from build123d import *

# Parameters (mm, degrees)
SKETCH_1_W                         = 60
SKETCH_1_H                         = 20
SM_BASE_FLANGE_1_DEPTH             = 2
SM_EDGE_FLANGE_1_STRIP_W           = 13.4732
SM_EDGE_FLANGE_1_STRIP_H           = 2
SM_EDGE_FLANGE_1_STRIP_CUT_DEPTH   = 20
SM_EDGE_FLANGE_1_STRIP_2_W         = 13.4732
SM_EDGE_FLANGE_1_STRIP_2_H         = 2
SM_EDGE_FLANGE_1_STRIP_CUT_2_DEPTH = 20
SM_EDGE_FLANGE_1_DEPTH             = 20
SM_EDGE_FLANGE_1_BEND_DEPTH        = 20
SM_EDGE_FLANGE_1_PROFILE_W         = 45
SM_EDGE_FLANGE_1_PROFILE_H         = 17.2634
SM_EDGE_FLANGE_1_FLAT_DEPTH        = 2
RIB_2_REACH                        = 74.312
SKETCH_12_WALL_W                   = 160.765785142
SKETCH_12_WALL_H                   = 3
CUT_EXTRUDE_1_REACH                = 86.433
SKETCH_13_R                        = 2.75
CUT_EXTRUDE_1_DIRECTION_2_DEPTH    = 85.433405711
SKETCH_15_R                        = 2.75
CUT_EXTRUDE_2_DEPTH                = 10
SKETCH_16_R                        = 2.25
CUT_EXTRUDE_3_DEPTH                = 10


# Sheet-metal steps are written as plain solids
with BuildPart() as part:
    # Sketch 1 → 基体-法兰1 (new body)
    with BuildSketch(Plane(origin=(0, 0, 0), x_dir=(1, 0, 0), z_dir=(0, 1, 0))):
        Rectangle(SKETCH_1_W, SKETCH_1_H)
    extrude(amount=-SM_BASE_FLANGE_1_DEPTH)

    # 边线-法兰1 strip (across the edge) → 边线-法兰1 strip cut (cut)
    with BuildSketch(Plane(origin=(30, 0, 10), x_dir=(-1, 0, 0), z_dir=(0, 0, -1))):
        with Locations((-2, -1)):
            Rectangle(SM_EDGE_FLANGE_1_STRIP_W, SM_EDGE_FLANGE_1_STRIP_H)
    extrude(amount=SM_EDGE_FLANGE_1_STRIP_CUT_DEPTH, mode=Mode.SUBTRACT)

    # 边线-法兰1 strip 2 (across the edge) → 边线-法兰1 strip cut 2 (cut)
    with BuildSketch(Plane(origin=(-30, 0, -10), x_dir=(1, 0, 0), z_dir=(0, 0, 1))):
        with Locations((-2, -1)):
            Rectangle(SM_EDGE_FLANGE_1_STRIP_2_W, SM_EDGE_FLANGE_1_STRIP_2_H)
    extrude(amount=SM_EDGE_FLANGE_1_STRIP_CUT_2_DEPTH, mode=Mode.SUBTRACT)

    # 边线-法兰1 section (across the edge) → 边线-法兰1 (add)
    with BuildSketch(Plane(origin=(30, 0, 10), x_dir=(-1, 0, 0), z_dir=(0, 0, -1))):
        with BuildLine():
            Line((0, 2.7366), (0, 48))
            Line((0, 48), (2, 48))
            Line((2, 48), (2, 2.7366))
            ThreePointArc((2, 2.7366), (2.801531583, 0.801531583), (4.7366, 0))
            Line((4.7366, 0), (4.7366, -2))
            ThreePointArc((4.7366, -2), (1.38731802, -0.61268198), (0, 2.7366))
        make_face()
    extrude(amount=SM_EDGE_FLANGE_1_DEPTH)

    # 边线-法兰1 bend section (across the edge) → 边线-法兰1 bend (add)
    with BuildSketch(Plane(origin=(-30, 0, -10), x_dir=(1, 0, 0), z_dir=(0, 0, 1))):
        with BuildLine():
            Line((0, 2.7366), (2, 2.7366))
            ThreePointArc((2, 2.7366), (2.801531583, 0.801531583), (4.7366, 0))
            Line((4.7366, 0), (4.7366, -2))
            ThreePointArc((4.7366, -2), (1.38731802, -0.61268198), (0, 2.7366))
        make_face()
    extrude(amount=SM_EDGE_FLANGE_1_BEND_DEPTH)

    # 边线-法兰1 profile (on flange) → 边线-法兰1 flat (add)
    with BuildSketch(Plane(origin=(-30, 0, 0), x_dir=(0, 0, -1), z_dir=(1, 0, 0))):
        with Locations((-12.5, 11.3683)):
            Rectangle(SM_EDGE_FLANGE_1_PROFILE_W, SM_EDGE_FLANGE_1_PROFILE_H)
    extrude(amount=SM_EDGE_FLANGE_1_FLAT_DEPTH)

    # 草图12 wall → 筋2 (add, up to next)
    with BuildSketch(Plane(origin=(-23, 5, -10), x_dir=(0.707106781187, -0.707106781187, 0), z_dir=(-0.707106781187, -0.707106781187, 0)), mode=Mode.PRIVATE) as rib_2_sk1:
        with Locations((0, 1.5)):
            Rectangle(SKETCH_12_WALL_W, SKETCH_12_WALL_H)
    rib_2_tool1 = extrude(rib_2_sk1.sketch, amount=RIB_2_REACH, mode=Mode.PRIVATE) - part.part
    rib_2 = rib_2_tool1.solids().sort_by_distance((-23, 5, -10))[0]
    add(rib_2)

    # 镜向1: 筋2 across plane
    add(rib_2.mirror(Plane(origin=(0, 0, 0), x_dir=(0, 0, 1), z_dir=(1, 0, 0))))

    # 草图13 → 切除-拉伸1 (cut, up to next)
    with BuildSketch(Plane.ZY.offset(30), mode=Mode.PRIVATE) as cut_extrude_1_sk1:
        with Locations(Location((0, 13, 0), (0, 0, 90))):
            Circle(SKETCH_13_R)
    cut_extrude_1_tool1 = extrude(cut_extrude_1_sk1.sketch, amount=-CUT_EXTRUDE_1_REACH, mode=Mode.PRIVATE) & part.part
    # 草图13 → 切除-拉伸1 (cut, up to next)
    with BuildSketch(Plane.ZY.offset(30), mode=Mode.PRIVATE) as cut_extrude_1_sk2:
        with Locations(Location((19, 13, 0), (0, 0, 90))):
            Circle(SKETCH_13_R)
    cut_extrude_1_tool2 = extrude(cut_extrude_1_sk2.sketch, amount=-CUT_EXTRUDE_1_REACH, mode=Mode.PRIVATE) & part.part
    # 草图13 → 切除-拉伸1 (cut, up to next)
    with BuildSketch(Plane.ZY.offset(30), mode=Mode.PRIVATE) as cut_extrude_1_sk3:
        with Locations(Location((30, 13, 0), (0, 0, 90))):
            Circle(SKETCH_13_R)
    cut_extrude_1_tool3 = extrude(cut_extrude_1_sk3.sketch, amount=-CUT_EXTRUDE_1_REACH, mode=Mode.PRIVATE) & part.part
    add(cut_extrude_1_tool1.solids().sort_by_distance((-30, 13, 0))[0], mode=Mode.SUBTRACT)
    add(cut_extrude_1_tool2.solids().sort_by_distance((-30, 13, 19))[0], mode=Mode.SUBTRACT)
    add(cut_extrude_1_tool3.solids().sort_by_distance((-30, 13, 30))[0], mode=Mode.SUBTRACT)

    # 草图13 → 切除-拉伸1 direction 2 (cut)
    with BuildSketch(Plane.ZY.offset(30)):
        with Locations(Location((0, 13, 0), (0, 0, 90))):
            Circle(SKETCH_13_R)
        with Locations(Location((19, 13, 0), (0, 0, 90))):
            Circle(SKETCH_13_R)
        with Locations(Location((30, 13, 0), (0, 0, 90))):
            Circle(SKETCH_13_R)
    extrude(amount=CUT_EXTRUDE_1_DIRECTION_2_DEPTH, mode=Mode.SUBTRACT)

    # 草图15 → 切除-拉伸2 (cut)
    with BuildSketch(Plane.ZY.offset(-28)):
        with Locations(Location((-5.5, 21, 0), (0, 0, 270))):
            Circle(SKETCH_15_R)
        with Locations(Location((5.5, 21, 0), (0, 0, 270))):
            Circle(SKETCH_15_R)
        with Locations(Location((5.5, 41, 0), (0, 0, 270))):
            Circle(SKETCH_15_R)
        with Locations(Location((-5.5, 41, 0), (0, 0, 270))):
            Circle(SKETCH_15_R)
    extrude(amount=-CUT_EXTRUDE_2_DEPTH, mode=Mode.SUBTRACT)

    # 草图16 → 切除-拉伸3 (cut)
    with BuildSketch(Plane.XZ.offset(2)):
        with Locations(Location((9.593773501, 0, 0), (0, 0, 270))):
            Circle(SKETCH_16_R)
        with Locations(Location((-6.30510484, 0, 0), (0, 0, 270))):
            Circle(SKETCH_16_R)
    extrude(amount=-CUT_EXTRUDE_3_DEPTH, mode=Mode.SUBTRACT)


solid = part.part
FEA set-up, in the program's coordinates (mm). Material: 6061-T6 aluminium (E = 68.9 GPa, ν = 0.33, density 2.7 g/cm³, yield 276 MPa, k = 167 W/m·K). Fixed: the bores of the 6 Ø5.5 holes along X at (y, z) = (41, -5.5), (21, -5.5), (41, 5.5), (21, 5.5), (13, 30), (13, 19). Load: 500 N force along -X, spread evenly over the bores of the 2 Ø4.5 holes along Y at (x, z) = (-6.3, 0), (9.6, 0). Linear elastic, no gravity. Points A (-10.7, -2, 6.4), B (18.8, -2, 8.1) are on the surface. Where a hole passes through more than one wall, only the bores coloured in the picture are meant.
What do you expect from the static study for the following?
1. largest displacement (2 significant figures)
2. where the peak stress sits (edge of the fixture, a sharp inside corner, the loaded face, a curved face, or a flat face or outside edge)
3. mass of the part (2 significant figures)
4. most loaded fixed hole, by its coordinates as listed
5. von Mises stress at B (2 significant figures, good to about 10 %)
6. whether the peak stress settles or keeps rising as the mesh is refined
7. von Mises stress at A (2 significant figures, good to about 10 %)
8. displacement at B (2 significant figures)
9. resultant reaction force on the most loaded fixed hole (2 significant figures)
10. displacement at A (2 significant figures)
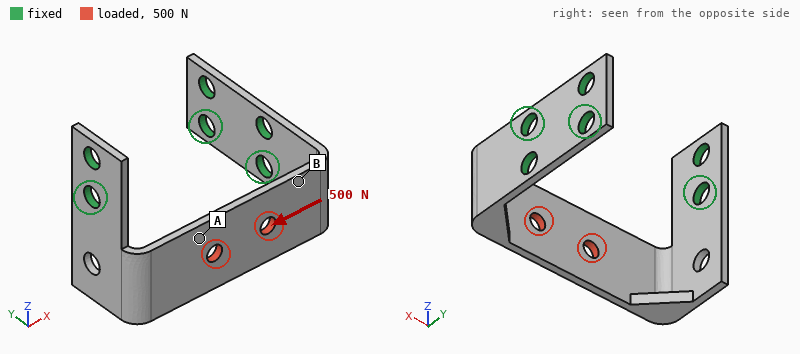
0.31 mm
edge of the fixture
16 g
(13, 19)
69 MPa
keeps rising
26 MPa
0.28 mm
320 N
0.25 mm
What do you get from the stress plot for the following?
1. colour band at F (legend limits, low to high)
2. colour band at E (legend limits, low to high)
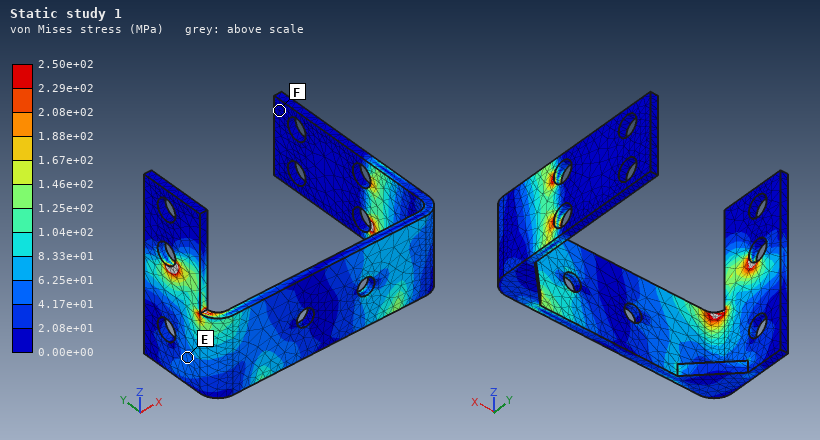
0.00e+00 to 2.08e+01 MPa
4.17e+01 to 6.25e+01 MPa
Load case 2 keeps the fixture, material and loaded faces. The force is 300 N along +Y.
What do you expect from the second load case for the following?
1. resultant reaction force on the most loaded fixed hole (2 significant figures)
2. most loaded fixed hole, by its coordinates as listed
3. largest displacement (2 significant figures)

260 N
(13, 19)
0.32 mm
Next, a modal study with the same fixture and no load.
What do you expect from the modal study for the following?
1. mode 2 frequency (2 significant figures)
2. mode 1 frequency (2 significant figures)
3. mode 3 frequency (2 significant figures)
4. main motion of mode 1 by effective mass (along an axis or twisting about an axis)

3000 Hz
2300 Hz
5400 Hz
along X
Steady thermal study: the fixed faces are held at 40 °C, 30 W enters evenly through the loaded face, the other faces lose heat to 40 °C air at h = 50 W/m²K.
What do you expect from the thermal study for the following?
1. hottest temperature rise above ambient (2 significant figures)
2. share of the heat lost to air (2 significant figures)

76 K
29 %
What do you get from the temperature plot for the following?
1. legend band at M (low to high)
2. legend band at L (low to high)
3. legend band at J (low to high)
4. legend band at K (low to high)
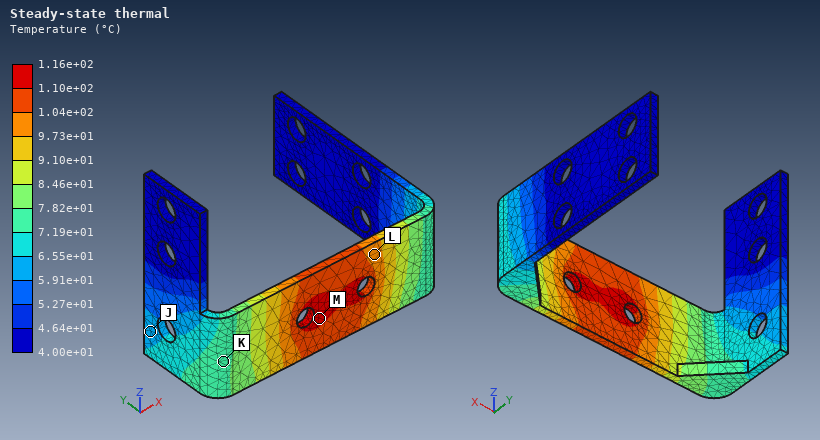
1.10e+02 to 1.16e+02 °C
9.73e+01 to 1.04e+02 °C
5.91e+01 to 6.55e+01 °C
7.19e+01 to 7.82e+01 °C
